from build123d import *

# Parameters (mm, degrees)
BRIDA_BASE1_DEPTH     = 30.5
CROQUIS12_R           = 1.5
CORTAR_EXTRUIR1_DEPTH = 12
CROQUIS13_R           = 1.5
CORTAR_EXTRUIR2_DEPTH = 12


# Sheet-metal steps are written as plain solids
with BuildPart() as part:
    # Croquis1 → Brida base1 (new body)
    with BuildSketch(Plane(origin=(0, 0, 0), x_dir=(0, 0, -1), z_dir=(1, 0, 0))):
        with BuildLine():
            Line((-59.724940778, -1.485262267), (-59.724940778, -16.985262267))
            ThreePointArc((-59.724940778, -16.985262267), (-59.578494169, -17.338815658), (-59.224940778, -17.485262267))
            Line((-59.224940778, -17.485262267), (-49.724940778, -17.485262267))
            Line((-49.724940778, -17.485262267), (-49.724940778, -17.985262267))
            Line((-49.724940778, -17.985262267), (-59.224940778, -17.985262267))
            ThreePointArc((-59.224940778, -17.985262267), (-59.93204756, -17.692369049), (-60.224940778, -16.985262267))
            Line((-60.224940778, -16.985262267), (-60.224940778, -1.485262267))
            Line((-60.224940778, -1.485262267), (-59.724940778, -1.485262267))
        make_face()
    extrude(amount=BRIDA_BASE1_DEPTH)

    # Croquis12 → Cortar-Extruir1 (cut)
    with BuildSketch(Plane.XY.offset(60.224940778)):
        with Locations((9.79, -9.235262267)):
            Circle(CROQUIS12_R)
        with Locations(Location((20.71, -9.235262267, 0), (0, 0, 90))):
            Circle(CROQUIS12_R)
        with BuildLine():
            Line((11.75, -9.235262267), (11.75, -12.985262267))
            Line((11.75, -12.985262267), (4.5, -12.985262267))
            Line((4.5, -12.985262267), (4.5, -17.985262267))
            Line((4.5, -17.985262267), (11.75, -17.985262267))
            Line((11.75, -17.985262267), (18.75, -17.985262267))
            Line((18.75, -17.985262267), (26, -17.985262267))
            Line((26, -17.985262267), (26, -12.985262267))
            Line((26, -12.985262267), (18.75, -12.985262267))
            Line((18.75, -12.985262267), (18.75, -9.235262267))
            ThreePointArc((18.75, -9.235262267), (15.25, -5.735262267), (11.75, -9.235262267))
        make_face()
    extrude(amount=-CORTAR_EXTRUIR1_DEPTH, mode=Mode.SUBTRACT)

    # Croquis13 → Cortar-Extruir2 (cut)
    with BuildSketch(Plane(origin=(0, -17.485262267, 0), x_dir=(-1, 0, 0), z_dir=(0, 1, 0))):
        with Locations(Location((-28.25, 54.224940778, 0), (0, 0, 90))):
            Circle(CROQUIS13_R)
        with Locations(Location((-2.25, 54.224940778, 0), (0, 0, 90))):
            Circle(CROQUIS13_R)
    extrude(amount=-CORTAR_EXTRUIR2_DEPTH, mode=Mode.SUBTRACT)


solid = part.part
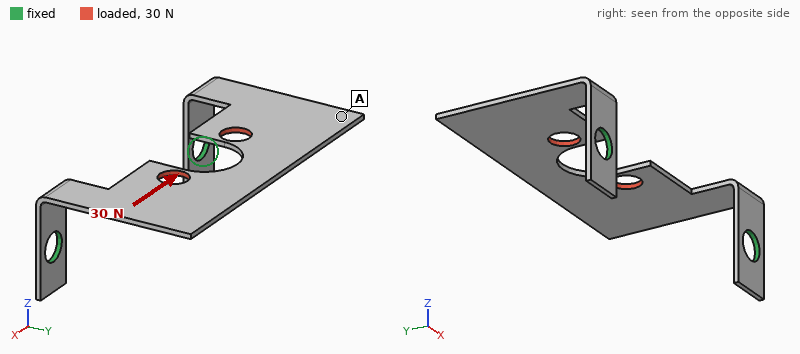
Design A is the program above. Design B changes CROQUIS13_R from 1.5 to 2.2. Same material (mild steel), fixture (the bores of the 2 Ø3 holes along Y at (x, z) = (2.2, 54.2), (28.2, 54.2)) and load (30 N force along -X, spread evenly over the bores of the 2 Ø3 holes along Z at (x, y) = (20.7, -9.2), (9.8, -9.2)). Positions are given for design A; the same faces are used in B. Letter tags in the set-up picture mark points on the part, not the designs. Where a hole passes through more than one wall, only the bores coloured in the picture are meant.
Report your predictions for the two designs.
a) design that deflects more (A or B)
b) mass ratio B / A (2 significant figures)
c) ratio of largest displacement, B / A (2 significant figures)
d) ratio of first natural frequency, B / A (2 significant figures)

A
0.96
0.71
1.1
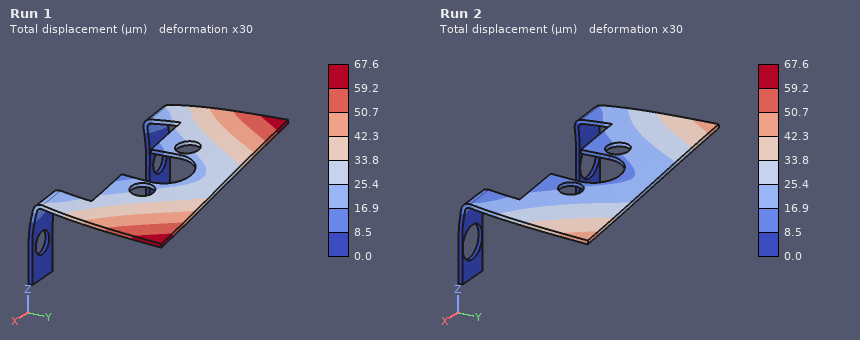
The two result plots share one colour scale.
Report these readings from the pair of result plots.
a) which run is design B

Run 2
